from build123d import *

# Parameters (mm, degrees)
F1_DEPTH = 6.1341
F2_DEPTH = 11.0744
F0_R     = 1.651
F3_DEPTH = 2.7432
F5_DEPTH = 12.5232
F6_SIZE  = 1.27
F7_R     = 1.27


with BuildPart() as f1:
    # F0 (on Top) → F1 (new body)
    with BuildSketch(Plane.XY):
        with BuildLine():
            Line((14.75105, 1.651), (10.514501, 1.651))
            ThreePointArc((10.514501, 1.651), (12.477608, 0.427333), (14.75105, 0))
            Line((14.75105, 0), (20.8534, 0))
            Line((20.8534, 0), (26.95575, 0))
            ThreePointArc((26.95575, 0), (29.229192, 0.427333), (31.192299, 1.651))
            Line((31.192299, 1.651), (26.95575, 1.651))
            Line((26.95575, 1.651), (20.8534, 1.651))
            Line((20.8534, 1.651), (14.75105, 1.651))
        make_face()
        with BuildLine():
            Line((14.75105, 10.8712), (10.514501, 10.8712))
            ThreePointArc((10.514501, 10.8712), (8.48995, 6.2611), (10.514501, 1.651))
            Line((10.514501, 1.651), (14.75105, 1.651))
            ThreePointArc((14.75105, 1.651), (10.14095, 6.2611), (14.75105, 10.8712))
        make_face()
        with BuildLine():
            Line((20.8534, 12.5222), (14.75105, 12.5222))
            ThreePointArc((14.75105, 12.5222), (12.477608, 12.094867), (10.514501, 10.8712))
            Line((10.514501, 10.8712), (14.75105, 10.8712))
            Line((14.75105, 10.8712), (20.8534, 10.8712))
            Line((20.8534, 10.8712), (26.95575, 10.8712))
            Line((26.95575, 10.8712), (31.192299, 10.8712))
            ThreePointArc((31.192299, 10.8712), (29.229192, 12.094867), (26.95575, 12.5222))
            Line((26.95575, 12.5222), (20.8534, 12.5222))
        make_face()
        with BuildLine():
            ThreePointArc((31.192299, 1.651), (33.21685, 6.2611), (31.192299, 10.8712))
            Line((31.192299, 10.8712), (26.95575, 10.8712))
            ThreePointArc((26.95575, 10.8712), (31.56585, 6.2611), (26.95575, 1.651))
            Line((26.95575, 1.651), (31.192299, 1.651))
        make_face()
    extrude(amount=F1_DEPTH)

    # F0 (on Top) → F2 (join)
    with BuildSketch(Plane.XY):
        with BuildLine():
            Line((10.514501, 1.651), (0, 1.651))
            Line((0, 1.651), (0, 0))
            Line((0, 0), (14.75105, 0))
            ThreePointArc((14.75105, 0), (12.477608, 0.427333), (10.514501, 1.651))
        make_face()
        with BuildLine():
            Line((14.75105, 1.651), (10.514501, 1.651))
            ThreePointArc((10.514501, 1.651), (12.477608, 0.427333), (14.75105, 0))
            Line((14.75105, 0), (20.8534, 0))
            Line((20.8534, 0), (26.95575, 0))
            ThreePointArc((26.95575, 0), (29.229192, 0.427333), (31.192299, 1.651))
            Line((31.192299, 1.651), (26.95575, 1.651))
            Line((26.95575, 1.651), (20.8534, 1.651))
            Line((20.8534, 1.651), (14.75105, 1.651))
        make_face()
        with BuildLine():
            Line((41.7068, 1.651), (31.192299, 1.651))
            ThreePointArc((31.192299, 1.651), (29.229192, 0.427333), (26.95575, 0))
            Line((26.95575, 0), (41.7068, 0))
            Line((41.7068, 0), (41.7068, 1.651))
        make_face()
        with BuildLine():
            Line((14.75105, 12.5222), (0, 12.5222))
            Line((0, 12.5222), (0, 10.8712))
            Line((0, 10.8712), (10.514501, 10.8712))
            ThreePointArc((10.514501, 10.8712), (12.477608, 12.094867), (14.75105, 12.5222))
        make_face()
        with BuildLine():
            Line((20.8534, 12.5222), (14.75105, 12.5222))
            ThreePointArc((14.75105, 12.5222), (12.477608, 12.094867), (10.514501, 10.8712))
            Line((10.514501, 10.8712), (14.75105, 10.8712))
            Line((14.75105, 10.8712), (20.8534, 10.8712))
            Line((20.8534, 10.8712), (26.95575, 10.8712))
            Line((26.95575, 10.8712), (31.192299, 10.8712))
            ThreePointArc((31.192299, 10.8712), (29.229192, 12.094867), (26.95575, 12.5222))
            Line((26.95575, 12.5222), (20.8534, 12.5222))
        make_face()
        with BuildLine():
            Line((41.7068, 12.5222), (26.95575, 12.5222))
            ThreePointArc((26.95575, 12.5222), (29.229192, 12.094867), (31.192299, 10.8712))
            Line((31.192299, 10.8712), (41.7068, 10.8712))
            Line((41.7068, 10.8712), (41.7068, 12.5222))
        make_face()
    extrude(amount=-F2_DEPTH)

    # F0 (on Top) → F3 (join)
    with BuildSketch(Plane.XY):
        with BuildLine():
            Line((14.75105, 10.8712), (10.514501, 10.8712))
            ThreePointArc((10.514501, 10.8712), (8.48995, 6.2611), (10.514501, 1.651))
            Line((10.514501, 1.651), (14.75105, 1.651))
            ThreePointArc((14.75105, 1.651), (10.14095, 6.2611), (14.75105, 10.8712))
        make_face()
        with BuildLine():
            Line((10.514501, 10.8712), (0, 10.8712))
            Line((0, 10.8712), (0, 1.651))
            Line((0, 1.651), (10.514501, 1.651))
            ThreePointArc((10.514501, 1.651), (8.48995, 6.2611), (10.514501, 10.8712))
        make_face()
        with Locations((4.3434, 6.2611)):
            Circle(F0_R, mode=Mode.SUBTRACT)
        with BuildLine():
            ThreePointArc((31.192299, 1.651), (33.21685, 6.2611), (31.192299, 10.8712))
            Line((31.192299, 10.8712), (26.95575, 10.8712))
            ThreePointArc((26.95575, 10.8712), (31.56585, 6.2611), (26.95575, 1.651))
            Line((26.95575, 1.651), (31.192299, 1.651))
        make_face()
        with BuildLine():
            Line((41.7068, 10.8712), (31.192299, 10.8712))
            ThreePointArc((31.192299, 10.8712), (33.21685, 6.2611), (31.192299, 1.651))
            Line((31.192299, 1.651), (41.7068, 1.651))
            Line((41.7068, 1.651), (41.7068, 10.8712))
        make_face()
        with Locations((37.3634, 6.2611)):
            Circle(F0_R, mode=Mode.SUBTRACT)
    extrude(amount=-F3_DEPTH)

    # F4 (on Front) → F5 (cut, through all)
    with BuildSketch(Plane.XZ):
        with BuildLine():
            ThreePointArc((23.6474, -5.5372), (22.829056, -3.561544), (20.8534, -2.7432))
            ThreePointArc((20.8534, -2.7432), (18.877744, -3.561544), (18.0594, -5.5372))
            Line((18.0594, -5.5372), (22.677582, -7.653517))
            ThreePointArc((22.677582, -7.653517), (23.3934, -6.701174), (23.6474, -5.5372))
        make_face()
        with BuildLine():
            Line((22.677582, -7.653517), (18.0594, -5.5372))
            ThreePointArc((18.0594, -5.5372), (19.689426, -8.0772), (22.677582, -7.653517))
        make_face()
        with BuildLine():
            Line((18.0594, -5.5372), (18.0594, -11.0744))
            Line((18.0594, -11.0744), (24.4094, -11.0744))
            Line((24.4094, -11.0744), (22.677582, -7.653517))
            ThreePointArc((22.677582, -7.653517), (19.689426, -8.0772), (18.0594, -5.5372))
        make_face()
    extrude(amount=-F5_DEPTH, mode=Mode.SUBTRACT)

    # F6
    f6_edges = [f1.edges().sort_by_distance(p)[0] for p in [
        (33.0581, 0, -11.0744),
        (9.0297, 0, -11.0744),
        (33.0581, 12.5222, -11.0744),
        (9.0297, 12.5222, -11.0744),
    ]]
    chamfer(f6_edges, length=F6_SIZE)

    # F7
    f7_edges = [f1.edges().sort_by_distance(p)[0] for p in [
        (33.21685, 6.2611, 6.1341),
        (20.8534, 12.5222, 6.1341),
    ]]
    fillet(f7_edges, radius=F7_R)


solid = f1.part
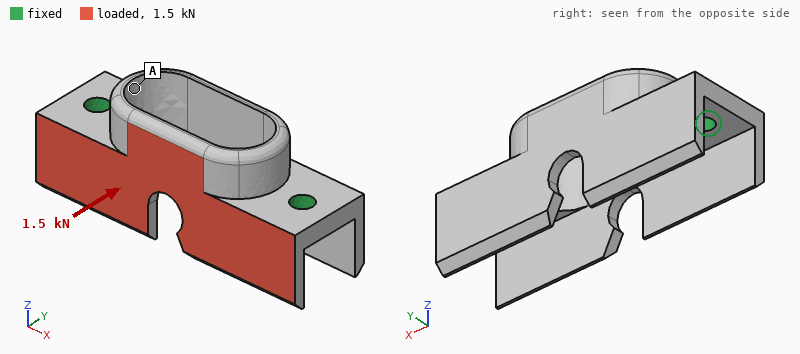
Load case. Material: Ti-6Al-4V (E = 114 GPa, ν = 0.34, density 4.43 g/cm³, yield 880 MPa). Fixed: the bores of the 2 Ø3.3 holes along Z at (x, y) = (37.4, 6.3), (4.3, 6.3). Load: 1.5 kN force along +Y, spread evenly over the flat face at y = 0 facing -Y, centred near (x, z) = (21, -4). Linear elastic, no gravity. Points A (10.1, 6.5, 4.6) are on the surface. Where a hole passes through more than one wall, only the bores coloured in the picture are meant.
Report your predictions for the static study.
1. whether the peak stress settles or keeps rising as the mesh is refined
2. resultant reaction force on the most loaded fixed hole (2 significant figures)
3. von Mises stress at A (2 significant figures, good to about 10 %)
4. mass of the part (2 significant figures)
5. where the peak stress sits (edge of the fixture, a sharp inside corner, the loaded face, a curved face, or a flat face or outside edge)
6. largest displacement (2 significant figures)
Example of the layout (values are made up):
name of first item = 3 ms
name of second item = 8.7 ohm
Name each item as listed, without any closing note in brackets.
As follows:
whether the peak stress settles or keeps rising as the mesh is refined = keeps rising
resultant reaction force on the most loaded fixed hole = 810 N
von Mises stress at A = 24 MPa
mass of the part = 11 g
where the peak stress sits = a sharp inside corner
largest displacement = 0.12 mm
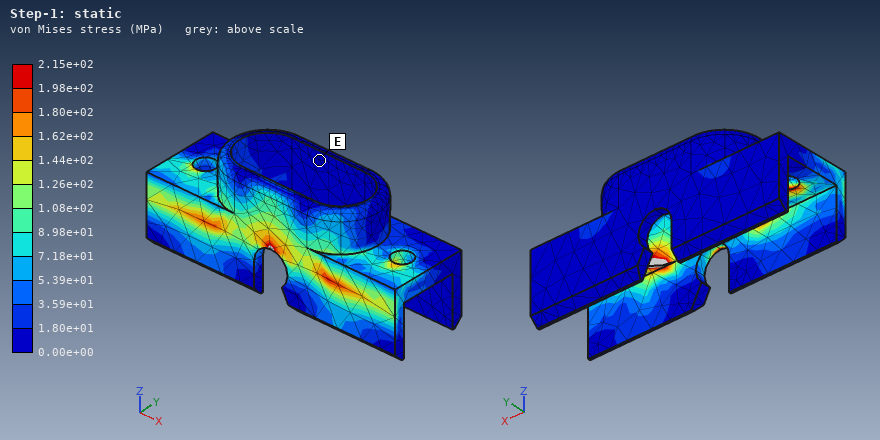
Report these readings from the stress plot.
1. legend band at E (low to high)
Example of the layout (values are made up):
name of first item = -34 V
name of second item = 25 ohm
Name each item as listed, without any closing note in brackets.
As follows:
legend band at E = 0.00e+00 to 1.80e+01 MPa
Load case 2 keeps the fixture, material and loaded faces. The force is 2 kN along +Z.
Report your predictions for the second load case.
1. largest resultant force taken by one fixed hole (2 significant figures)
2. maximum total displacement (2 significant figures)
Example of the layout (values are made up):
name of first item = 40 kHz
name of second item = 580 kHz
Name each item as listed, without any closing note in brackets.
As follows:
largest resultant force taken by one fixed hole = 1.0 kN
maximum total displacement = 0.11 mm
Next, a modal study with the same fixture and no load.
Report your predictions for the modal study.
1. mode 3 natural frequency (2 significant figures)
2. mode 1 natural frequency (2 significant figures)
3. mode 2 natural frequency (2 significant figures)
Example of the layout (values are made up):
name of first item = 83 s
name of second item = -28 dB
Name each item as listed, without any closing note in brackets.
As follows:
mode 3 natural frequency = 13 kHz
mode 1 natural frequency = 11 kHz
mode 2 natural frequency = 13 kHz
